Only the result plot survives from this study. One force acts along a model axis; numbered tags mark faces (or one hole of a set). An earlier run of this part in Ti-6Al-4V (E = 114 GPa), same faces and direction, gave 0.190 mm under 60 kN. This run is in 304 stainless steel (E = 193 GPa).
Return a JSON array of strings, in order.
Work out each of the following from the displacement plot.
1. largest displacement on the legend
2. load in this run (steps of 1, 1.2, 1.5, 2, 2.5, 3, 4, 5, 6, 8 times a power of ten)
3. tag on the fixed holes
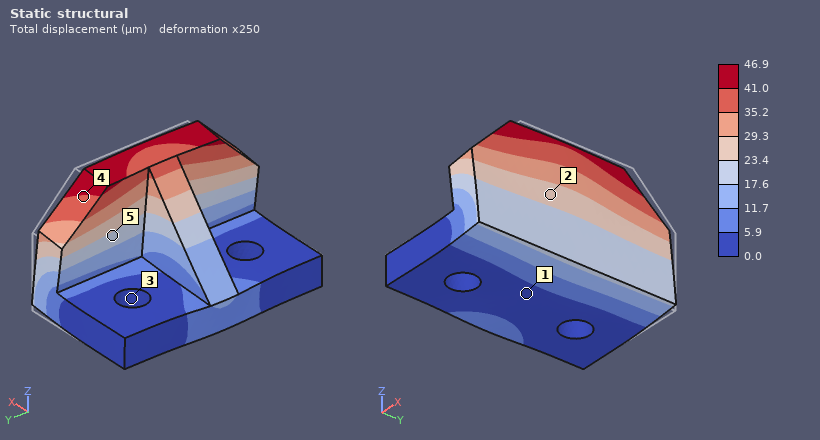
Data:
["46.9 µm", "25 kN", "3"]
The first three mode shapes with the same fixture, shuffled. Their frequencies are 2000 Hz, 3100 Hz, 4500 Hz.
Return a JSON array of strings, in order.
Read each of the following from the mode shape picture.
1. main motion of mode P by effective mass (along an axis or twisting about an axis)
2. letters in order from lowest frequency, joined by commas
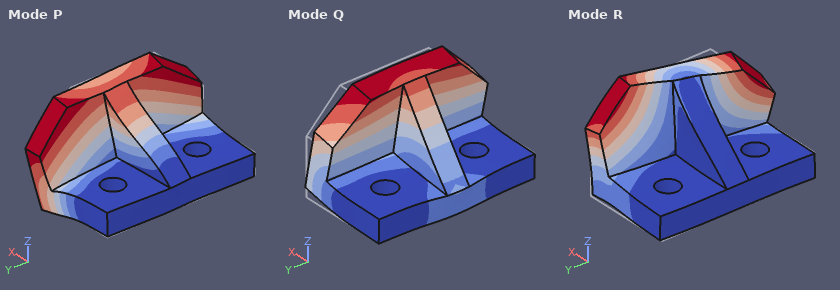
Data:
["along Y", "Q, P, R"]
